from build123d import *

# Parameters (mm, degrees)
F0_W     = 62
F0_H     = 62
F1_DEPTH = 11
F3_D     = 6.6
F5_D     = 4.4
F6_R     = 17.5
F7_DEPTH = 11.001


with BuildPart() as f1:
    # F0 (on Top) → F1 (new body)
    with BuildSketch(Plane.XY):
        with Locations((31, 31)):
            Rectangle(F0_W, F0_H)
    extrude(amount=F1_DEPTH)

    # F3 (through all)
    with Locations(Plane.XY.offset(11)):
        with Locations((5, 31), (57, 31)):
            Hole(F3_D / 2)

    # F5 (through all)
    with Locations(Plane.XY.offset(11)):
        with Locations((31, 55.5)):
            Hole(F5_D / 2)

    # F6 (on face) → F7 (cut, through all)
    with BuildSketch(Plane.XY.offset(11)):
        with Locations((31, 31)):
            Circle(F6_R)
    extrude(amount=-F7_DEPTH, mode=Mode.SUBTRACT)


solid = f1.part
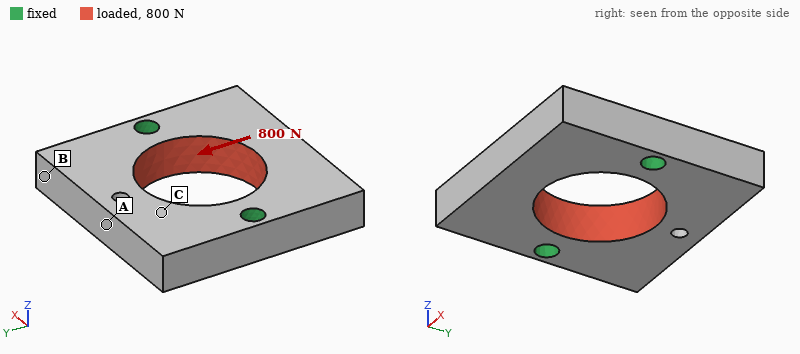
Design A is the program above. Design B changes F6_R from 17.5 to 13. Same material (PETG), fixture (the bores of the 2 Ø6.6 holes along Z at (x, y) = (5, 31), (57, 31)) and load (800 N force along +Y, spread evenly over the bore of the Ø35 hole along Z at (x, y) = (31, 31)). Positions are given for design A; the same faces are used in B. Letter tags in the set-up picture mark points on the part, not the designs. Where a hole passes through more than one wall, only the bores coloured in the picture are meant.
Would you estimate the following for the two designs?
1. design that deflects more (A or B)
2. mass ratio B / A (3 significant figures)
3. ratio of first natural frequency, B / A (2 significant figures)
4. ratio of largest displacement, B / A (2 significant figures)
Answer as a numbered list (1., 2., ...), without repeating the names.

1. A
2. 1.15
3. 1.0
4. 0.90
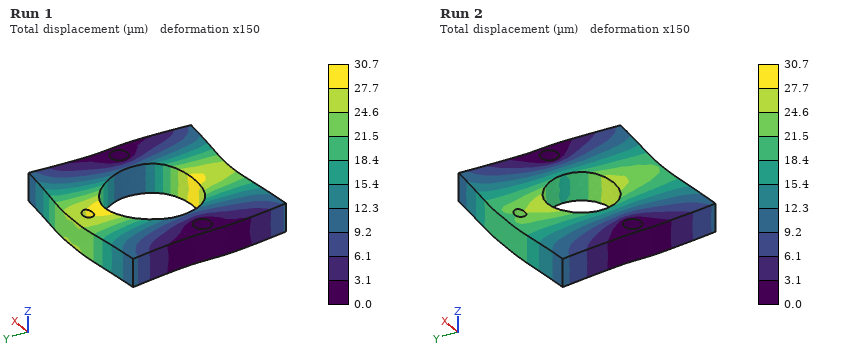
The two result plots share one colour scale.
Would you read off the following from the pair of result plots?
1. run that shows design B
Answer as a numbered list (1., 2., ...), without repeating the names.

1. Run 2
